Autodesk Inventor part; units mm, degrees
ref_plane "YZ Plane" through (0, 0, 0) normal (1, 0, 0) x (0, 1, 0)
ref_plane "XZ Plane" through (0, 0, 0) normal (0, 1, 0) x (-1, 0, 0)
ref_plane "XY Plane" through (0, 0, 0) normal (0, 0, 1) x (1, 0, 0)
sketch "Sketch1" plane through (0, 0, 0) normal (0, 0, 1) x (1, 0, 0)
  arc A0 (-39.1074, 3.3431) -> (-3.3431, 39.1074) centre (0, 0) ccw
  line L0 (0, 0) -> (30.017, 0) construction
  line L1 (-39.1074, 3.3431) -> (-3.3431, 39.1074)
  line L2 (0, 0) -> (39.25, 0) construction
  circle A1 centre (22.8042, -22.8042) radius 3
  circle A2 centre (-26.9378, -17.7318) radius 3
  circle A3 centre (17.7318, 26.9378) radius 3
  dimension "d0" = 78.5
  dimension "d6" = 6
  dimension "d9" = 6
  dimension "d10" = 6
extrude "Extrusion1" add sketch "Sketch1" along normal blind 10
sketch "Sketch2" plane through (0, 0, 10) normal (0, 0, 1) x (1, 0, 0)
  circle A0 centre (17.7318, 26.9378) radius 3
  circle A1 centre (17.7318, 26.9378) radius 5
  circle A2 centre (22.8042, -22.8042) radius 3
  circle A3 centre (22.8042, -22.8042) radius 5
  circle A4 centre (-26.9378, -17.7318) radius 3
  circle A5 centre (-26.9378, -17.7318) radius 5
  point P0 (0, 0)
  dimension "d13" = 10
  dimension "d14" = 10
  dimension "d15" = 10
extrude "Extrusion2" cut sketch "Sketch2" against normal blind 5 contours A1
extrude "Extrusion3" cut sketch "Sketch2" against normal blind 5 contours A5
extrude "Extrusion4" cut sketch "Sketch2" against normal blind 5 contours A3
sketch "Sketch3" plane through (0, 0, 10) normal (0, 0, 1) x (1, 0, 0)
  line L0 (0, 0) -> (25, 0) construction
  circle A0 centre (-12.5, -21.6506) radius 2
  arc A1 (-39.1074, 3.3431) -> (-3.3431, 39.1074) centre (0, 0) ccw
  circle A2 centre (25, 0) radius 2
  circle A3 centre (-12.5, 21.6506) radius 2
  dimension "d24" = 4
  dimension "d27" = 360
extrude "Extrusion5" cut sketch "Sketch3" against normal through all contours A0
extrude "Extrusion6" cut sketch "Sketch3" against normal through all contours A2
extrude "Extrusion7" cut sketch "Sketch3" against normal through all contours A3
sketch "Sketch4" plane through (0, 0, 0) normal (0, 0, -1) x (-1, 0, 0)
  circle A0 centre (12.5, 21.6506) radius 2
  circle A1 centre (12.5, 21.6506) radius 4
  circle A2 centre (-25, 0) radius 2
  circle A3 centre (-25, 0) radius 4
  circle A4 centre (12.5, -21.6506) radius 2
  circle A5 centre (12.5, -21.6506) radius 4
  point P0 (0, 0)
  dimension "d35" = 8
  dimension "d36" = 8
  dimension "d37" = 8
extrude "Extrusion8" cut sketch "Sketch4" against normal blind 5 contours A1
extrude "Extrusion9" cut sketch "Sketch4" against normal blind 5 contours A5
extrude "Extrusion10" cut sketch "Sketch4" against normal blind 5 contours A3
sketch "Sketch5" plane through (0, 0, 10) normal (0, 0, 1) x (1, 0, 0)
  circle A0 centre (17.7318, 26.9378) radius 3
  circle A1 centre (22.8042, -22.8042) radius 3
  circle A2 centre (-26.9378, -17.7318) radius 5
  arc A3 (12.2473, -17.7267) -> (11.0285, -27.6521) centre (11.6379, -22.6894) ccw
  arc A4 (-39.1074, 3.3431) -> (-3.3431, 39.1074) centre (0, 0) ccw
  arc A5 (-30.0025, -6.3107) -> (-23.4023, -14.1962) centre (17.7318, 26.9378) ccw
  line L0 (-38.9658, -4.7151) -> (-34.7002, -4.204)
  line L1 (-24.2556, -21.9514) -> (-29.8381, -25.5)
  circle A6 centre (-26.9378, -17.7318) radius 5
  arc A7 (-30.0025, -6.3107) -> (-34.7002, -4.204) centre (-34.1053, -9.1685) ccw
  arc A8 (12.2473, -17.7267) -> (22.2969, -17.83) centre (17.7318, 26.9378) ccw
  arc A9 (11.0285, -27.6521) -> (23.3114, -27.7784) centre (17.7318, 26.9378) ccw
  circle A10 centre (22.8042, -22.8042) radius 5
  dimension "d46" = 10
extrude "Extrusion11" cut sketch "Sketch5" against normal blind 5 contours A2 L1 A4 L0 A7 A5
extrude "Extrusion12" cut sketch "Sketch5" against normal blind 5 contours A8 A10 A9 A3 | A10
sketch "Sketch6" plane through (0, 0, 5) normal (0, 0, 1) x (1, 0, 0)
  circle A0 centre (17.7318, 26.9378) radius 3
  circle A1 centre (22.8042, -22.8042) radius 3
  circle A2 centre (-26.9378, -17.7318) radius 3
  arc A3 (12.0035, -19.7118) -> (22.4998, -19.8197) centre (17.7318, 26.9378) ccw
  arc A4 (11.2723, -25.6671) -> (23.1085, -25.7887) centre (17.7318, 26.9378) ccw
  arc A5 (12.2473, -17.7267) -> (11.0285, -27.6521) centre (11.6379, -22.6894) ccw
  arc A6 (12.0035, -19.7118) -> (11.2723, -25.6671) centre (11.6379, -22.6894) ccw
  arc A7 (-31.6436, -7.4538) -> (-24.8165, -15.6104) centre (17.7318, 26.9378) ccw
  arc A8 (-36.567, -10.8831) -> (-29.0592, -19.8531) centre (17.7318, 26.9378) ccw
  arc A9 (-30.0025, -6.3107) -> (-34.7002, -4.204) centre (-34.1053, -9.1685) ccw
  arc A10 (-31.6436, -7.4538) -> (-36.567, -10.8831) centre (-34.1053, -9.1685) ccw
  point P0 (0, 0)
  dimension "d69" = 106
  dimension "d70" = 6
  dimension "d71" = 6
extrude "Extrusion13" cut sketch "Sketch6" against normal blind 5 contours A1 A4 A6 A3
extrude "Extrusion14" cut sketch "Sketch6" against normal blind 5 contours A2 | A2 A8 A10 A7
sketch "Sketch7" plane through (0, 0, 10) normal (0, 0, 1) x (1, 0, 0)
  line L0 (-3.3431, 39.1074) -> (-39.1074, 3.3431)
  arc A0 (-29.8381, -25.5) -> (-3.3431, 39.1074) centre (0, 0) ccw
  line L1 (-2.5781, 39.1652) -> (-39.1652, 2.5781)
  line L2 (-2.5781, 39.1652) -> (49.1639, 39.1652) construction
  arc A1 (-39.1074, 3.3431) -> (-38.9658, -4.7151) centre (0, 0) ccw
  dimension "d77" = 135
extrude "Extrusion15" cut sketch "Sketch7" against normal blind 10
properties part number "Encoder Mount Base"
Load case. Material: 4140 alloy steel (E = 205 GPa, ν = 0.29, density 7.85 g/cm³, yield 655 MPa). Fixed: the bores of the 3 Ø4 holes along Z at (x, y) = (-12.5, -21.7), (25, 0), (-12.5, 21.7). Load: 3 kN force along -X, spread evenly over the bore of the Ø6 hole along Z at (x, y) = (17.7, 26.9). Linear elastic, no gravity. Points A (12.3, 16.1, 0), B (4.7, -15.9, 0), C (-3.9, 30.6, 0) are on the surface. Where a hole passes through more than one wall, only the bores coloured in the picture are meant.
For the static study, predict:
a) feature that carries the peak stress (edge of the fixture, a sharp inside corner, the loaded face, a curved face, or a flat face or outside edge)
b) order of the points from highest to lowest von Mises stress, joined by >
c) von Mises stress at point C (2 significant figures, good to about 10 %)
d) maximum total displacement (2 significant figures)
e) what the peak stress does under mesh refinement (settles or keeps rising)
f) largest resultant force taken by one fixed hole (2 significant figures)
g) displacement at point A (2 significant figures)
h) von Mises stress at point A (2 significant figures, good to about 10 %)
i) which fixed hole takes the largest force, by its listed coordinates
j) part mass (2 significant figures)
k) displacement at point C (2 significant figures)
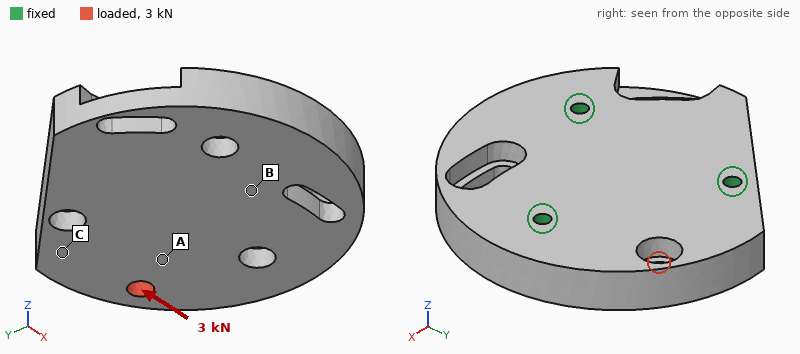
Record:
edge of the fixture
A > C > B
9.4 MPa
5.8 µm
keeps rising
2.0 kN
2.0 µm
16 MPa
(-12.5, 21.7)
320 g
2.2 µm
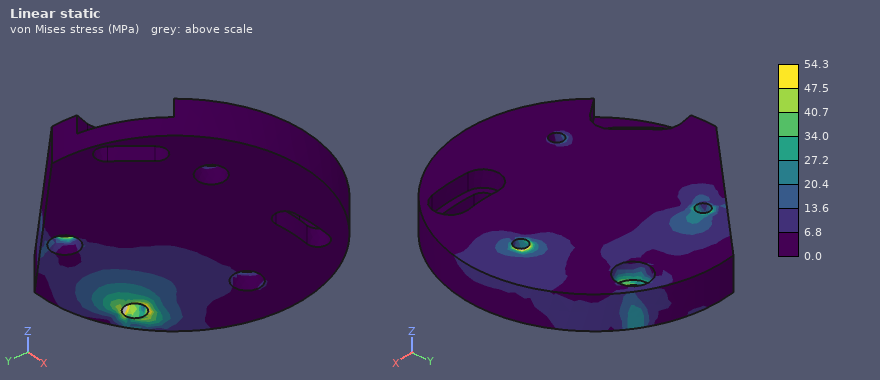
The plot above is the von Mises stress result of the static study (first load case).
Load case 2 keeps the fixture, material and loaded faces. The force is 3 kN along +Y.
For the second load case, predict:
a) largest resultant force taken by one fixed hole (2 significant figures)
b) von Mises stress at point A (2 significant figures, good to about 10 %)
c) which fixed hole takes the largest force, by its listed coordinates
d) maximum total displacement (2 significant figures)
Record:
1.8 kN
22 MPa
(25, 0)
8.7 µm
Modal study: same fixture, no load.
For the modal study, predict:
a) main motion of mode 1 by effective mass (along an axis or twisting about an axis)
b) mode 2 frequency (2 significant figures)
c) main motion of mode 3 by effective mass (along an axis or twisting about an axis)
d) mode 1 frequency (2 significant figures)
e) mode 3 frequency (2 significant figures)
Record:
twisting about X
7900 Hz
along Z
7200 Hz
11 kHz
